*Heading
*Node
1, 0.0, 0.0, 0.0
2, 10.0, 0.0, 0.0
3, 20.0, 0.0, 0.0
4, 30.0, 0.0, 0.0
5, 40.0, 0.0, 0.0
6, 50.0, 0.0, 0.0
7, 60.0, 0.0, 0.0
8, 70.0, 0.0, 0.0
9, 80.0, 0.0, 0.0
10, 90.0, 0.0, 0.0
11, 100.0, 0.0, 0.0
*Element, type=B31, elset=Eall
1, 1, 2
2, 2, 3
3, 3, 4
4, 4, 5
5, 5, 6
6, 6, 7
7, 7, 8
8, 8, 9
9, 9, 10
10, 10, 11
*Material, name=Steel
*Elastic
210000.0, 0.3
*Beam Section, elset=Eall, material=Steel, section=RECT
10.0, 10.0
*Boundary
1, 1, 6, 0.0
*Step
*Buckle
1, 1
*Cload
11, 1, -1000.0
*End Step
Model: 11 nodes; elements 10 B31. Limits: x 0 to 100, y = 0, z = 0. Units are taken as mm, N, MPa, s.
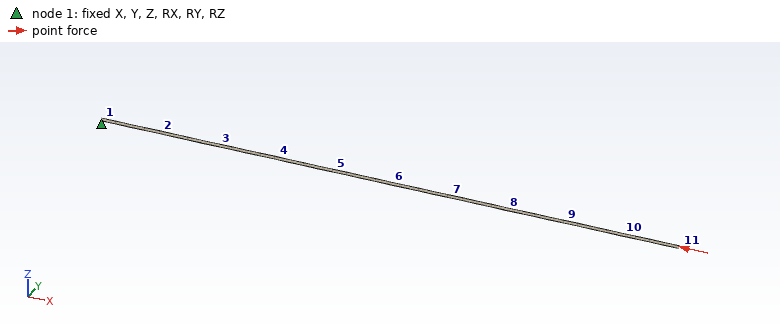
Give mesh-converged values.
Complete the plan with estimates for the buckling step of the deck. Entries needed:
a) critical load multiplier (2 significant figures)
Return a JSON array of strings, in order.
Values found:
["43"]
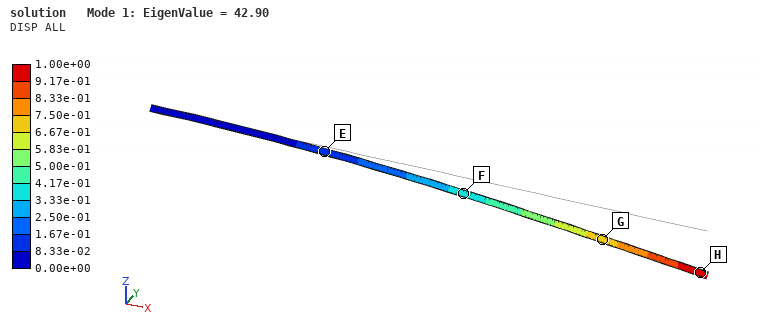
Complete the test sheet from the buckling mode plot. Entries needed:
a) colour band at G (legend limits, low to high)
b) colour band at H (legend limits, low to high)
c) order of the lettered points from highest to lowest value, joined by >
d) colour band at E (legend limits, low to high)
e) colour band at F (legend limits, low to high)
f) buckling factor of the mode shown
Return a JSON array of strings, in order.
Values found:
["6.67e-01 to 7.50e-01", "9.17e-01 to 1.00e+00", "H > G > F > E", "8.33e-02 to 1.67e-01", "3.33e-01 to 4.17e-01", "42.90"]
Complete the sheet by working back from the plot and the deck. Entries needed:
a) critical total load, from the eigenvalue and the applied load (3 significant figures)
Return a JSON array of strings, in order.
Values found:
["42900 N"]
